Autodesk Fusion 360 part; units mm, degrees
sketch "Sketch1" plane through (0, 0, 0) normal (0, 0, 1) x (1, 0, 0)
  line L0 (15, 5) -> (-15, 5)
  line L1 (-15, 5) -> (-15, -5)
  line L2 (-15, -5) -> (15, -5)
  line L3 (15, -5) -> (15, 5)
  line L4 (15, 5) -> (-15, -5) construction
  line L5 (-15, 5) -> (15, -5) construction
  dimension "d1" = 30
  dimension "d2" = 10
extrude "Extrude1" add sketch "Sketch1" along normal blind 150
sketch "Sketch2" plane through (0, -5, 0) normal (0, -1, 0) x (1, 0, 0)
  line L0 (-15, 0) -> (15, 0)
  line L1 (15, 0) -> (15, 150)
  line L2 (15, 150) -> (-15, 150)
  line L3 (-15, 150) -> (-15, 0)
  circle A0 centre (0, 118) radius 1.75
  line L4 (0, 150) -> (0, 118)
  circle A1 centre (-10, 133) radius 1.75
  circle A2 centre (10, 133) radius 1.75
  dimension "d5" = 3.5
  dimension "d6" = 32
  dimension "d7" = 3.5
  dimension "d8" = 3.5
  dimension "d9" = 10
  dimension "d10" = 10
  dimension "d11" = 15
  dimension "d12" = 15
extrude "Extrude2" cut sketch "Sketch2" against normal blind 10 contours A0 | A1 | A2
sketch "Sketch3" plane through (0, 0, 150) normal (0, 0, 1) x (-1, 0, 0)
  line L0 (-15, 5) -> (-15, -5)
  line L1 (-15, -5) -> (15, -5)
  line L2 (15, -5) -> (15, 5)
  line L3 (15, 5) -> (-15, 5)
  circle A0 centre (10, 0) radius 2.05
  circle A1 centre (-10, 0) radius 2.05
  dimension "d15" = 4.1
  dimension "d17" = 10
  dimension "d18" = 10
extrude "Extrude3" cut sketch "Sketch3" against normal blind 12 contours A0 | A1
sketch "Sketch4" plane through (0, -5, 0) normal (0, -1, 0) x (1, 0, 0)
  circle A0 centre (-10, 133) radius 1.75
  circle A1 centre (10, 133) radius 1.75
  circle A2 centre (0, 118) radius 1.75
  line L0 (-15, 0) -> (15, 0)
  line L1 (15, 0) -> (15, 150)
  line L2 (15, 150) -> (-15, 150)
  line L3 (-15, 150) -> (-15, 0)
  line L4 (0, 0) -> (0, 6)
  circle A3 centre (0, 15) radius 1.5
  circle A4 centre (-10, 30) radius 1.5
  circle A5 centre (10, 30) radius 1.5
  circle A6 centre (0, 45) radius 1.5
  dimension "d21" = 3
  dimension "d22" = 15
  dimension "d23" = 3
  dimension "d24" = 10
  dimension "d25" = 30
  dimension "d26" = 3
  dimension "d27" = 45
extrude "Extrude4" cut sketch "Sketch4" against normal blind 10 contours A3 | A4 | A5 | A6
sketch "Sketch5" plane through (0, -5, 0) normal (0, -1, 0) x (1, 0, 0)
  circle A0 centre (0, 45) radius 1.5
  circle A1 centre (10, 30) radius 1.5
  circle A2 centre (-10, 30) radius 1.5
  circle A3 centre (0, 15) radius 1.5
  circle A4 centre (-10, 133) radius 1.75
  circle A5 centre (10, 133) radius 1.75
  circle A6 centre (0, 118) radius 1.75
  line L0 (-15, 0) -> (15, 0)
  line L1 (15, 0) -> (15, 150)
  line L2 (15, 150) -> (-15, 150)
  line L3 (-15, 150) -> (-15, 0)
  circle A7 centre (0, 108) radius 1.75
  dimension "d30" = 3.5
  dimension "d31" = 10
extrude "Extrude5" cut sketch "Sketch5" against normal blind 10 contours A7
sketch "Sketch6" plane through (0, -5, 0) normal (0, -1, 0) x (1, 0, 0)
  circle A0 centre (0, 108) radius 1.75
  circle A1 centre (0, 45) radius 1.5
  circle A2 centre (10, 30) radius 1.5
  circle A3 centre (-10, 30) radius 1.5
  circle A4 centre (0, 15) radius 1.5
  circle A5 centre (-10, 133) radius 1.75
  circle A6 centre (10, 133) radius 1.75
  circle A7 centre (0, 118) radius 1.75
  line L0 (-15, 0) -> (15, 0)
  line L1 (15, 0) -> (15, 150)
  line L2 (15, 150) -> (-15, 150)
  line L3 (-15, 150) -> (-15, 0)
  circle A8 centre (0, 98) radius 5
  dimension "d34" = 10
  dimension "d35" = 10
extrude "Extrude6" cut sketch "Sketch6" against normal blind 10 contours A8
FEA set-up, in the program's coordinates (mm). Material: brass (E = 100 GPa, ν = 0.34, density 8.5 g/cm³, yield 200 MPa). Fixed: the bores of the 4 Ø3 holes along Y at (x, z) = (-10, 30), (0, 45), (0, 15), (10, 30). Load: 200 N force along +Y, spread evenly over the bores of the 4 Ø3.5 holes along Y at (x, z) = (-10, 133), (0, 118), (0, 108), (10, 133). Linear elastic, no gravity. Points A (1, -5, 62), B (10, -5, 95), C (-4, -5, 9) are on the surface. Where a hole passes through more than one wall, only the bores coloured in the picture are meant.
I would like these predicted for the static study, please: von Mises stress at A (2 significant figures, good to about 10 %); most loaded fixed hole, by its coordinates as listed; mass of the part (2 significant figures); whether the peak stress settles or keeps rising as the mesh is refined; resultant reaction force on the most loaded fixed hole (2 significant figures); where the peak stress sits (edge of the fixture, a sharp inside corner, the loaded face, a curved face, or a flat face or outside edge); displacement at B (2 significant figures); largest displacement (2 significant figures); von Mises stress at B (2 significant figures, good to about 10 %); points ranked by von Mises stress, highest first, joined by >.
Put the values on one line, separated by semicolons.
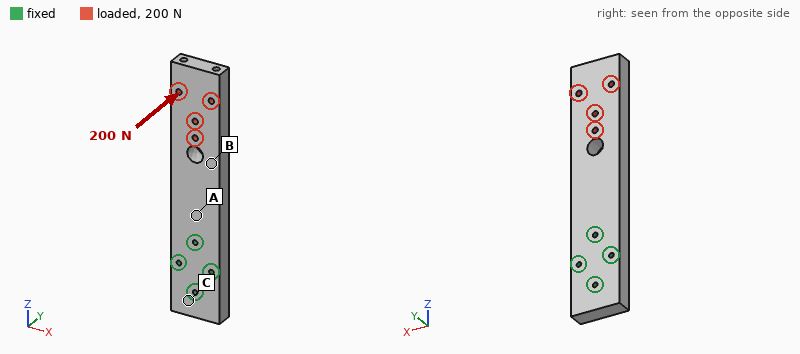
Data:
23 MPa; (0, 45); 370 g; keeps rising; 710 N; edge of the fixture; 0.072 mm; 0.22 mm; 15 MPa; A > B > C
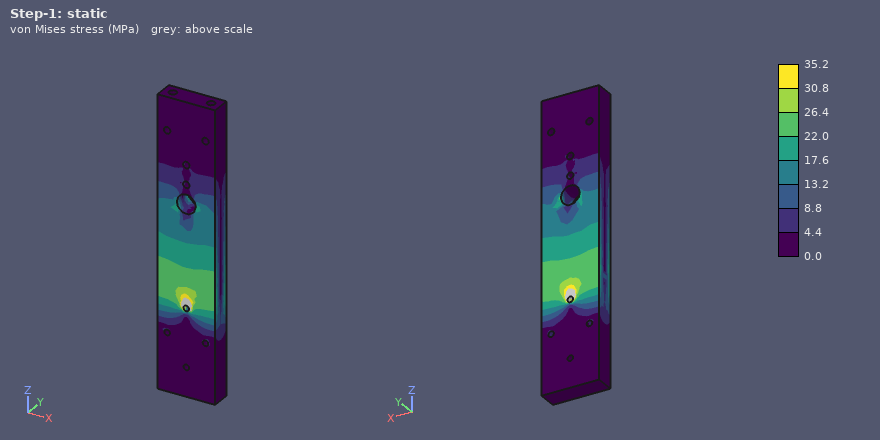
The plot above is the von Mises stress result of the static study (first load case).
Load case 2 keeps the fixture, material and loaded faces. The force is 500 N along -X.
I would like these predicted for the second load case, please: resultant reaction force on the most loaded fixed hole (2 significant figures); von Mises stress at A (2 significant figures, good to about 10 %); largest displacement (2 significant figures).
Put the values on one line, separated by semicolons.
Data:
1.3 kN; 4.2 MPa; 84 µm
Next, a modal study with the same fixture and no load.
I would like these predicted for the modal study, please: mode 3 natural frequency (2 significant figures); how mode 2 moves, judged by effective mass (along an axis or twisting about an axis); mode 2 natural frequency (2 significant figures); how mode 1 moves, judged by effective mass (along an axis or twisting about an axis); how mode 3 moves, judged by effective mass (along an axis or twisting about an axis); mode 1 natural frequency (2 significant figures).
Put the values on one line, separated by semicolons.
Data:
2700 Hz; along X; 1200 Hz; along Y; twisting about Z; 490 Hz
